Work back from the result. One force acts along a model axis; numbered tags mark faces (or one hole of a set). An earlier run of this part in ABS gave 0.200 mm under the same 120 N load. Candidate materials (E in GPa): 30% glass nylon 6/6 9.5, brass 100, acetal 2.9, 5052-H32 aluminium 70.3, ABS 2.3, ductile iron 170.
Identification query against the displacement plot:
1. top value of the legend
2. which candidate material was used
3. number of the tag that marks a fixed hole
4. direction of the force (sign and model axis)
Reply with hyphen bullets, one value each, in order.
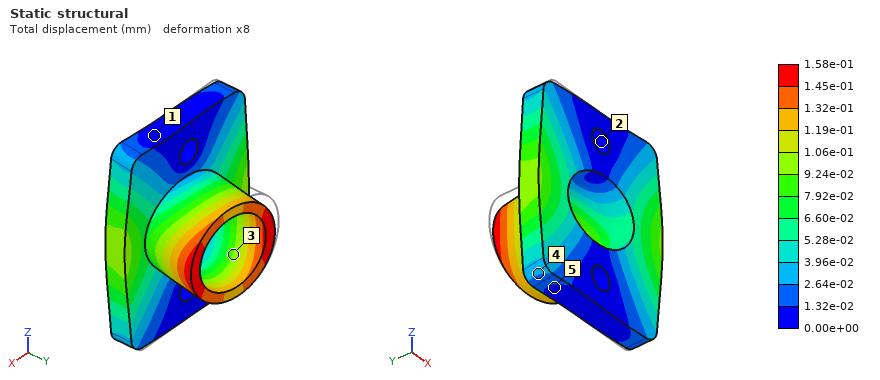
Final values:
- 1.58e-01 mm
- acetal
- 2
- +X
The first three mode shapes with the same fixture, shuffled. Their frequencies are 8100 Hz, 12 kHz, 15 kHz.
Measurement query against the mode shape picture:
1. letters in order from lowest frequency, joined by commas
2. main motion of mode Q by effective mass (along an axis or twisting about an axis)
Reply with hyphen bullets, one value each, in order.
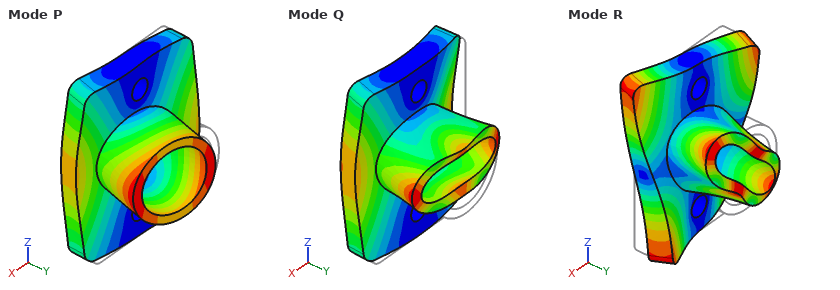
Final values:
- P, Q, R
- along Y
